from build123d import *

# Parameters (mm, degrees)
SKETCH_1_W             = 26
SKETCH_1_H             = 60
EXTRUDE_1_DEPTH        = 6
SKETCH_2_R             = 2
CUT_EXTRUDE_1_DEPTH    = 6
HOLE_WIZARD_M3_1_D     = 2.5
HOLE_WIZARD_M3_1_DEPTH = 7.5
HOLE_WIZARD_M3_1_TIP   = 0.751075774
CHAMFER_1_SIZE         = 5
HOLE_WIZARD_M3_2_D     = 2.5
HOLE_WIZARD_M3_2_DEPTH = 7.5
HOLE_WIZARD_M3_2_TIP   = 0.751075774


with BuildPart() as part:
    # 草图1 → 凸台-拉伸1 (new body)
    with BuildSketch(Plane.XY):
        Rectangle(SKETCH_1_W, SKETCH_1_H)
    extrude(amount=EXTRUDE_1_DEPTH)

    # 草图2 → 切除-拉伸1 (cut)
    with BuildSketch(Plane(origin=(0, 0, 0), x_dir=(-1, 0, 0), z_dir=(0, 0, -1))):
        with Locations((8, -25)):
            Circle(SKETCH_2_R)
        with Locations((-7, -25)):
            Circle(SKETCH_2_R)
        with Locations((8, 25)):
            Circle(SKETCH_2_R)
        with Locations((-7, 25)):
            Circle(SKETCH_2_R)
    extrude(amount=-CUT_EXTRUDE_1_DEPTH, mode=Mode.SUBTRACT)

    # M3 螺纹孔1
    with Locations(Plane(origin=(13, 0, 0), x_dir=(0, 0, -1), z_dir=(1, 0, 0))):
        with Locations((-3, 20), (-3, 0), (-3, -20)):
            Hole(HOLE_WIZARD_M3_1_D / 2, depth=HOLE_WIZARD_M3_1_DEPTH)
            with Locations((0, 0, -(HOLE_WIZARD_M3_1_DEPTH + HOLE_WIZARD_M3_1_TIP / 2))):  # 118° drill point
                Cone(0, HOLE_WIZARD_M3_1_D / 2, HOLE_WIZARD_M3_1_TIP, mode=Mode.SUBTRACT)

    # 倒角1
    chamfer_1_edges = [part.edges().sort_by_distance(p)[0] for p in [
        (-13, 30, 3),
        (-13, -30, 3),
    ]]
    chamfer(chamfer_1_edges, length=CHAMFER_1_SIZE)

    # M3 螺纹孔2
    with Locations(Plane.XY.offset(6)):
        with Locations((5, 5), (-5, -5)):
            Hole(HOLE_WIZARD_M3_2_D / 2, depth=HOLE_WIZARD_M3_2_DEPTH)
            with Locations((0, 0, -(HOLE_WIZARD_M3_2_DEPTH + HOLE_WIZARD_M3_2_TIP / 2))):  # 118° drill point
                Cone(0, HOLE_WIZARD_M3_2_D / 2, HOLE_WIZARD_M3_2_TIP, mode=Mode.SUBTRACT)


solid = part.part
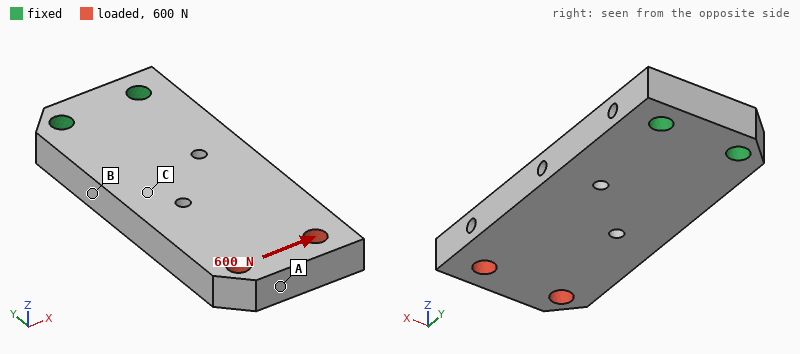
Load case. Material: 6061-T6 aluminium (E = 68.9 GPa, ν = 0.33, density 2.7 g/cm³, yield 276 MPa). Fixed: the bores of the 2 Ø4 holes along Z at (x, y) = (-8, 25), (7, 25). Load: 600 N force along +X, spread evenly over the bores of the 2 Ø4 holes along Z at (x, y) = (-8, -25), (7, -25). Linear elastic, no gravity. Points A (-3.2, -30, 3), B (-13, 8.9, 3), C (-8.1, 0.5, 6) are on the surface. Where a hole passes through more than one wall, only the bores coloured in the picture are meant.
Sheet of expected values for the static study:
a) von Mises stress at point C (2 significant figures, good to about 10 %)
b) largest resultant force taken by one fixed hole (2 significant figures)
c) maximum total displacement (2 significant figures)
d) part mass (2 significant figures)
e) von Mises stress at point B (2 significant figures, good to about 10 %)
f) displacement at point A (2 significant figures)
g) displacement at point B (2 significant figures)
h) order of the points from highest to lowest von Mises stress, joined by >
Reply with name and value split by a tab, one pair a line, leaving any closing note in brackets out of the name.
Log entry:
von Mises stress at point C	15 MPa
largest resultant force taken by one fixed hole	1.7 kN
maximum total displacement	67 µm
part mass	24 g
von Mises stress at point B	31 MPa
displacement at point A	64 µm
displacement at point B	15 µm
order of the points from highest to lowest von Mises stress, joined by >	B > C > A
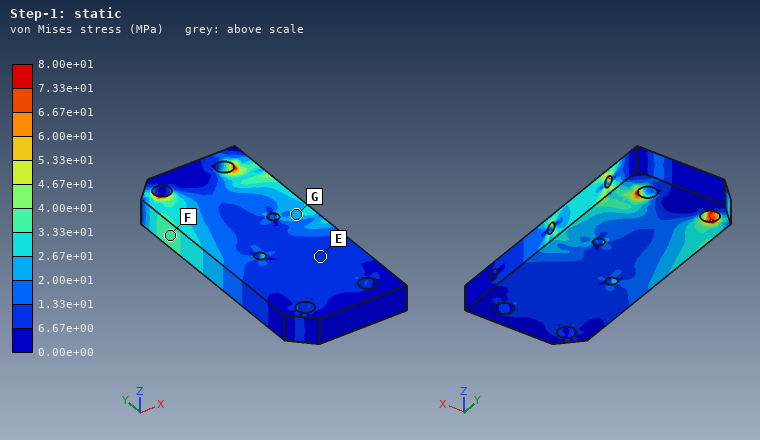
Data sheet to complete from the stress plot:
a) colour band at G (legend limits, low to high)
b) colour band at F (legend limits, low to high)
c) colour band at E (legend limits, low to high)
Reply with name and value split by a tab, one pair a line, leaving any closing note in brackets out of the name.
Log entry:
colour band at G	2.00e+01 to 2.67e+01 MPa
colour band at F	3.33e+01 to 4.00e+01 MPa
colour band at E	6.67e+00 to 1.33e+01 MPa
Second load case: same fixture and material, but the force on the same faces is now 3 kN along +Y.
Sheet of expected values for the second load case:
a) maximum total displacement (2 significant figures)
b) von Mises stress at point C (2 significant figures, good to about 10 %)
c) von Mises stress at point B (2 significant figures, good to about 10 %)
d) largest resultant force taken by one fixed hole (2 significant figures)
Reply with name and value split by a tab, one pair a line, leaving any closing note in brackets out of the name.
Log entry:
maximum total displacement	19 µm
von Mises stress at point C	21 MPa
von Mises stress at point B	20 MPa
largest resultant force taken by one fixed hole	1.5 kN
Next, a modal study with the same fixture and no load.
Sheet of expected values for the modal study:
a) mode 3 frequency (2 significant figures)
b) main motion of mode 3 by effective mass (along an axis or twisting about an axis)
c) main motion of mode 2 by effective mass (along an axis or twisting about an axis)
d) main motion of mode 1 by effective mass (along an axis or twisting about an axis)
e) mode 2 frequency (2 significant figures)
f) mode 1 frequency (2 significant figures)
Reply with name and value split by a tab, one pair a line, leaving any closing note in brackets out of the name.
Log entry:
mode 3 frequency	6800 Hz
main motion of mode 3 by effective mass	twisting about Y
main motion of mode 2 by effective mass	along X
main motion of mode 1 by effective mass	along Z
mode 2 frequency	5900 Hz
mode 1 frequency	1700 Hz
